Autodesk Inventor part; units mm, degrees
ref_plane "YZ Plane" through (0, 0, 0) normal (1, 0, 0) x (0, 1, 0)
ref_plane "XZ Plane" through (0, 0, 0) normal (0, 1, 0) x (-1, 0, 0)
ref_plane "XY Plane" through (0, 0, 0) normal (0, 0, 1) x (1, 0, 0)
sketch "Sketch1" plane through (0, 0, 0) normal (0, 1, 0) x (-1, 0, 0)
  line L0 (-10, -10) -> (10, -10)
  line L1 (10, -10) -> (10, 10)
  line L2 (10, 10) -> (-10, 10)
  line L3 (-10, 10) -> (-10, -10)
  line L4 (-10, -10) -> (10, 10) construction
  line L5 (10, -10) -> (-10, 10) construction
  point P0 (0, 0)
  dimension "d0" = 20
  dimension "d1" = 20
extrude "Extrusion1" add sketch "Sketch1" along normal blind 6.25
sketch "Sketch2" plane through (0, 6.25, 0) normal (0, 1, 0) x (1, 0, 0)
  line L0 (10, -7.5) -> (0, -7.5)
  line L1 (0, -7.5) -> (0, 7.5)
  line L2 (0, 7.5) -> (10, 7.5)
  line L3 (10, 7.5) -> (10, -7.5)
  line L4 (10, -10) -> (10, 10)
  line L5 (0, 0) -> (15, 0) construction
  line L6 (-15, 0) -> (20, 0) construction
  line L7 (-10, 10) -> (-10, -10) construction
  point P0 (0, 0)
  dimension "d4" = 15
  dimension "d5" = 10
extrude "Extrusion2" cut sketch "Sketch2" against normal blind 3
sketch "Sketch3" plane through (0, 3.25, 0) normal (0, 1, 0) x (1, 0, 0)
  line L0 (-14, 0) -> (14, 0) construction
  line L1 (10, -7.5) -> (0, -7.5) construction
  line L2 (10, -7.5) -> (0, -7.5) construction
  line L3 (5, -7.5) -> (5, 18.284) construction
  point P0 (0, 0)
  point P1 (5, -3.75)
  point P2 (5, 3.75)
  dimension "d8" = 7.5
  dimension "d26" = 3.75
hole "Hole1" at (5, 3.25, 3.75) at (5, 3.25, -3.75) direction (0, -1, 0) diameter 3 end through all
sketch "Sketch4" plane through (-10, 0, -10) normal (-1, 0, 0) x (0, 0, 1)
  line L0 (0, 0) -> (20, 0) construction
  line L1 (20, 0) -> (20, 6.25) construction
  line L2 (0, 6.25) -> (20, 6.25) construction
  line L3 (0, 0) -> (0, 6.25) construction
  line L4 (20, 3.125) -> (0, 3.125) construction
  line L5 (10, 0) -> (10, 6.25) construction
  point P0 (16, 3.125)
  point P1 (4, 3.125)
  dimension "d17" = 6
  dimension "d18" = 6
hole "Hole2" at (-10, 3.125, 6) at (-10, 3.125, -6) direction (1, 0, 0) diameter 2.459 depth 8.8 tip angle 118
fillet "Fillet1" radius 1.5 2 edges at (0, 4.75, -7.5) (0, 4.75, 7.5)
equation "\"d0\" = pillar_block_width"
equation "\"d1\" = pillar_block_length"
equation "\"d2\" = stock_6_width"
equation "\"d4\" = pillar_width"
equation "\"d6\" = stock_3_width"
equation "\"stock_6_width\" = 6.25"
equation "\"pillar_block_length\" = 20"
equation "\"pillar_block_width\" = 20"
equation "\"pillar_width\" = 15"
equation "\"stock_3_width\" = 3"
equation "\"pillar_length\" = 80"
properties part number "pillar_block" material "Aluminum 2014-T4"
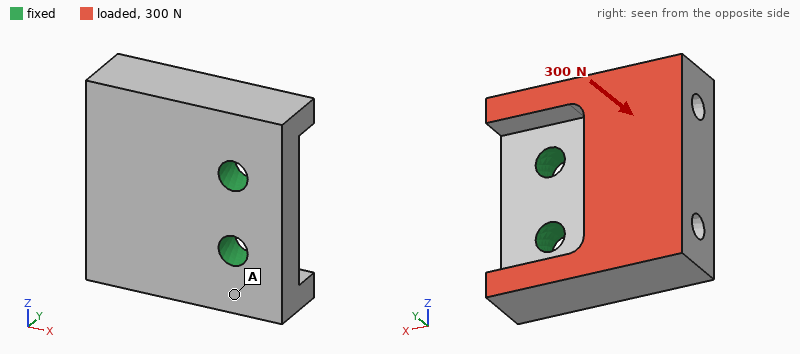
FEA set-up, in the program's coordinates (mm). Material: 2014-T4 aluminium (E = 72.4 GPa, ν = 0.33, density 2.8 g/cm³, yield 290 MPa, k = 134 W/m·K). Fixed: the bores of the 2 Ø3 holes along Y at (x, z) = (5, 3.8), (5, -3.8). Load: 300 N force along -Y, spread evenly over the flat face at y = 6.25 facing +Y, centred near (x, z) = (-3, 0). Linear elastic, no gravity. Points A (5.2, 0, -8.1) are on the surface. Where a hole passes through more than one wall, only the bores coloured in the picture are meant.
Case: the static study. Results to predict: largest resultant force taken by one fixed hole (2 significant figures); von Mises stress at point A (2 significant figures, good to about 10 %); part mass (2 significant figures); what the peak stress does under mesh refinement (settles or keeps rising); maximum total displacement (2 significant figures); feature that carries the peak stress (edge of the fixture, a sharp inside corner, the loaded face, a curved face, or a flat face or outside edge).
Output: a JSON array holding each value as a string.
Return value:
["150 N", "15 MPa", "5.4 g", "keeps rising", "21 µm", "edge of the fixture"]
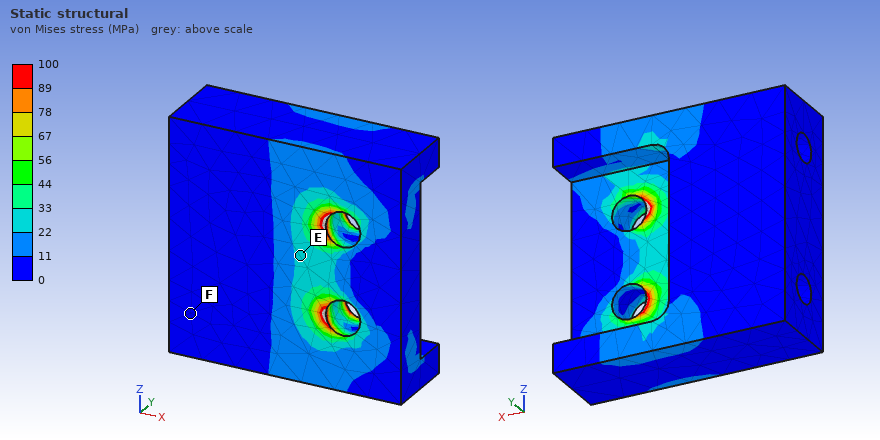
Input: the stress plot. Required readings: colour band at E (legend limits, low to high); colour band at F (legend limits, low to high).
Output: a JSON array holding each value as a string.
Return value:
["22 to 33 MPa", "0 to 11 MPa"]
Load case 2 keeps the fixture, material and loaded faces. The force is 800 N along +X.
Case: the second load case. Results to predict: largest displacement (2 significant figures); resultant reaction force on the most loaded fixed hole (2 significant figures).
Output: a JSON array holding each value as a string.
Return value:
["40 µm", "400 N"]
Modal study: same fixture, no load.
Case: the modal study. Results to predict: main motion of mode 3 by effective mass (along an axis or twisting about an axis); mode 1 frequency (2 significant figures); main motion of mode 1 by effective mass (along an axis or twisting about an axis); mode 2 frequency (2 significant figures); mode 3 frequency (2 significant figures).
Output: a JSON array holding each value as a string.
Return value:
["along Z", "11 kHz", "along Y", "21 kHz", "24 kHz"]
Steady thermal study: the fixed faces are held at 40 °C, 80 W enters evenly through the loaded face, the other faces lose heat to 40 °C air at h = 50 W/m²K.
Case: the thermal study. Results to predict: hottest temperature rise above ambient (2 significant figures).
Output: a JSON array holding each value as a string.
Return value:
["68 K"]
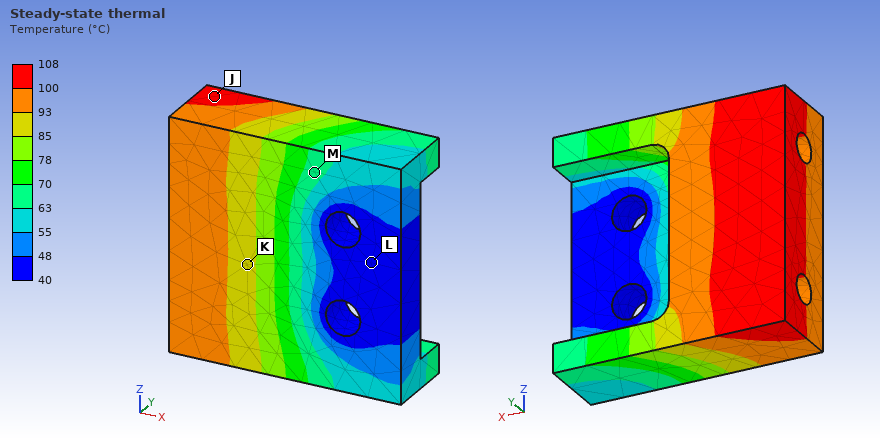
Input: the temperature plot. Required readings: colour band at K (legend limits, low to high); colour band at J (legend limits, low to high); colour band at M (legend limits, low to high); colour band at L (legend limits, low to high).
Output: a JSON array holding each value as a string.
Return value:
["85 to 93 °C", "100 to 108 °C", "63 to 70 °C", "40 to 48 °C"]
